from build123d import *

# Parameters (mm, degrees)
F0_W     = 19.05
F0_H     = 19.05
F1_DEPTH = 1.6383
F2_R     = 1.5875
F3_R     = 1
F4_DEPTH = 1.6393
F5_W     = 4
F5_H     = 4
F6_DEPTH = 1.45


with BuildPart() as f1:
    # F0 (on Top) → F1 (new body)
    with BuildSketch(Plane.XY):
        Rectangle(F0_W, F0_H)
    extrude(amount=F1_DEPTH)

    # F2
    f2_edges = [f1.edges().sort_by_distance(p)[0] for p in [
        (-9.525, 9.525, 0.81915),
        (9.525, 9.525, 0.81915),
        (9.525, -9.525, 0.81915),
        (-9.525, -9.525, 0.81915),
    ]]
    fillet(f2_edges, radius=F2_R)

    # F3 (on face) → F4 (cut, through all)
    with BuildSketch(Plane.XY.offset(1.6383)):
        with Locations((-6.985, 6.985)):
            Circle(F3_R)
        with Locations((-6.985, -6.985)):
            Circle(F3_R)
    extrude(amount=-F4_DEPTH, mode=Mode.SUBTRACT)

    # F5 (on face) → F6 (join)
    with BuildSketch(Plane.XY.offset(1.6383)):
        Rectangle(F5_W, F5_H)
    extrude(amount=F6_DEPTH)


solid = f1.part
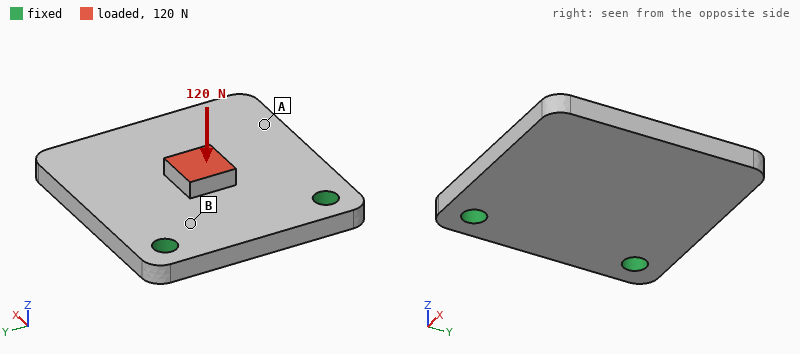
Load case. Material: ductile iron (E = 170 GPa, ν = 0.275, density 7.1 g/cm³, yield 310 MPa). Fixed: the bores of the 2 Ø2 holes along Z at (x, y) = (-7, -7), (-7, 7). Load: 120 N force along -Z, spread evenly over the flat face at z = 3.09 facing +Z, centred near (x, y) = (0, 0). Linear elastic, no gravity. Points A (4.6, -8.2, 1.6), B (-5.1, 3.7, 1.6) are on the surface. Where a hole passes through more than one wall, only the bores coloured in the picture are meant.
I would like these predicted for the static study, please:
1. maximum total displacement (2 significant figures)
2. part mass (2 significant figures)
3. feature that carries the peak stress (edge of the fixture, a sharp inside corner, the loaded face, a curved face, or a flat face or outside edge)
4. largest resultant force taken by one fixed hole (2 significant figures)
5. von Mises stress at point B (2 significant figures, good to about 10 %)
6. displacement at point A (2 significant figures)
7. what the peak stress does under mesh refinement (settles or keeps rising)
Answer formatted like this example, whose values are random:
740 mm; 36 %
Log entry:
44 µm; 4.3 g; edge of the fixture; 60 N; 56 MPa; 26 µm; keeps rising
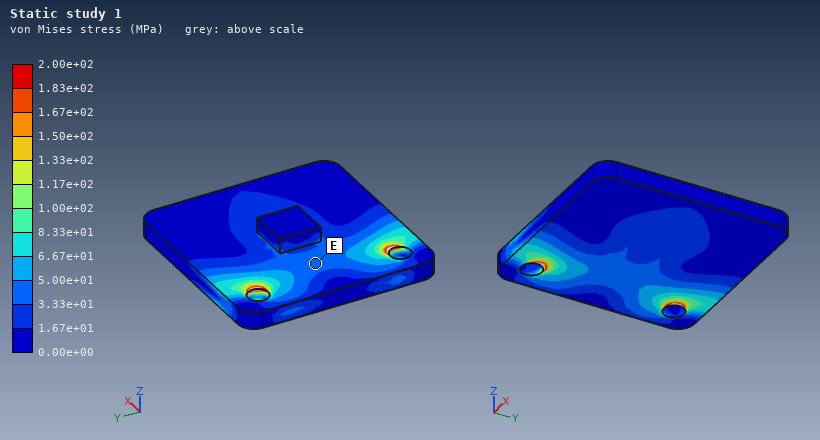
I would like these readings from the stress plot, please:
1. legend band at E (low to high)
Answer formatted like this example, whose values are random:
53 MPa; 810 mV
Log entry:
3.33e+01 to 5.00e+01 MPa
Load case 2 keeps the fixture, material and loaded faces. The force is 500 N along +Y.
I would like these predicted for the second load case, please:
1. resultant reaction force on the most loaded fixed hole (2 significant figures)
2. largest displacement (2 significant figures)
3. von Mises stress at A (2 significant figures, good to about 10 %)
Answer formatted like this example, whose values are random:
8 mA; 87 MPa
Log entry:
350 N; 17 µm; 25 MPa
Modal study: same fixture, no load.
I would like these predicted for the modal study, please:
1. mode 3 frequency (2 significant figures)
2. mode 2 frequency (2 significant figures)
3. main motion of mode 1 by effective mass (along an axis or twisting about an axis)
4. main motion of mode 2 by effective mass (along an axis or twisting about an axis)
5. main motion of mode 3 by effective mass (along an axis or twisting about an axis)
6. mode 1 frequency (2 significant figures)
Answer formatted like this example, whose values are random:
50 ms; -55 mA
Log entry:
27 kHz; 11 kHz; along Z; twisting about X; along Z; 4600 Hz
